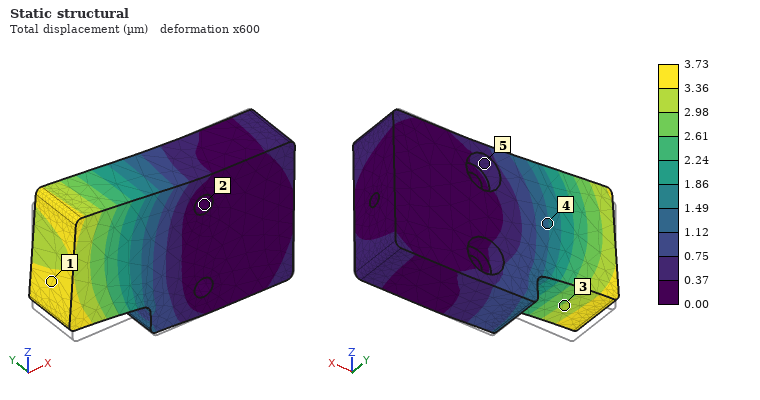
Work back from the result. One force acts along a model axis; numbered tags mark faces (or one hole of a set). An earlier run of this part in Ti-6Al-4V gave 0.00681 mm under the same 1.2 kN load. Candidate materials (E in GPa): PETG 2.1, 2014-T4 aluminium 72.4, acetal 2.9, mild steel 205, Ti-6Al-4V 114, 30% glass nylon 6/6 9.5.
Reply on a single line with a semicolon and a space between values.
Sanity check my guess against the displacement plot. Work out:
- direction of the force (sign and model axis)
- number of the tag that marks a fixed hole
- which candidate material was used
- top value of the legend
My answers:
+Z; 2; mild steel; 3.73 µm
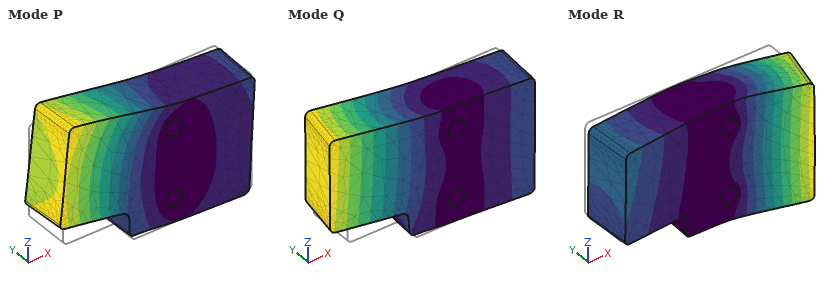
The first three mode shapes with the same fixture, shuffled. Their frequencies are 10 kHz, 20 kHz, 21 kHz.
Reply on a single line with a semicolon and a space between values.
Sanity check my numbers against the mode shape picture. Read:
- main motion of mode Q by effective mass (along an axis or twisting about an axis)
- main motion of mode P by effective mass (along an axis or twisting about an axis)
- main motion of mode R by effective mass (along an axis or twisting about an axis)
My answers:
along Y; along Z; along Y
